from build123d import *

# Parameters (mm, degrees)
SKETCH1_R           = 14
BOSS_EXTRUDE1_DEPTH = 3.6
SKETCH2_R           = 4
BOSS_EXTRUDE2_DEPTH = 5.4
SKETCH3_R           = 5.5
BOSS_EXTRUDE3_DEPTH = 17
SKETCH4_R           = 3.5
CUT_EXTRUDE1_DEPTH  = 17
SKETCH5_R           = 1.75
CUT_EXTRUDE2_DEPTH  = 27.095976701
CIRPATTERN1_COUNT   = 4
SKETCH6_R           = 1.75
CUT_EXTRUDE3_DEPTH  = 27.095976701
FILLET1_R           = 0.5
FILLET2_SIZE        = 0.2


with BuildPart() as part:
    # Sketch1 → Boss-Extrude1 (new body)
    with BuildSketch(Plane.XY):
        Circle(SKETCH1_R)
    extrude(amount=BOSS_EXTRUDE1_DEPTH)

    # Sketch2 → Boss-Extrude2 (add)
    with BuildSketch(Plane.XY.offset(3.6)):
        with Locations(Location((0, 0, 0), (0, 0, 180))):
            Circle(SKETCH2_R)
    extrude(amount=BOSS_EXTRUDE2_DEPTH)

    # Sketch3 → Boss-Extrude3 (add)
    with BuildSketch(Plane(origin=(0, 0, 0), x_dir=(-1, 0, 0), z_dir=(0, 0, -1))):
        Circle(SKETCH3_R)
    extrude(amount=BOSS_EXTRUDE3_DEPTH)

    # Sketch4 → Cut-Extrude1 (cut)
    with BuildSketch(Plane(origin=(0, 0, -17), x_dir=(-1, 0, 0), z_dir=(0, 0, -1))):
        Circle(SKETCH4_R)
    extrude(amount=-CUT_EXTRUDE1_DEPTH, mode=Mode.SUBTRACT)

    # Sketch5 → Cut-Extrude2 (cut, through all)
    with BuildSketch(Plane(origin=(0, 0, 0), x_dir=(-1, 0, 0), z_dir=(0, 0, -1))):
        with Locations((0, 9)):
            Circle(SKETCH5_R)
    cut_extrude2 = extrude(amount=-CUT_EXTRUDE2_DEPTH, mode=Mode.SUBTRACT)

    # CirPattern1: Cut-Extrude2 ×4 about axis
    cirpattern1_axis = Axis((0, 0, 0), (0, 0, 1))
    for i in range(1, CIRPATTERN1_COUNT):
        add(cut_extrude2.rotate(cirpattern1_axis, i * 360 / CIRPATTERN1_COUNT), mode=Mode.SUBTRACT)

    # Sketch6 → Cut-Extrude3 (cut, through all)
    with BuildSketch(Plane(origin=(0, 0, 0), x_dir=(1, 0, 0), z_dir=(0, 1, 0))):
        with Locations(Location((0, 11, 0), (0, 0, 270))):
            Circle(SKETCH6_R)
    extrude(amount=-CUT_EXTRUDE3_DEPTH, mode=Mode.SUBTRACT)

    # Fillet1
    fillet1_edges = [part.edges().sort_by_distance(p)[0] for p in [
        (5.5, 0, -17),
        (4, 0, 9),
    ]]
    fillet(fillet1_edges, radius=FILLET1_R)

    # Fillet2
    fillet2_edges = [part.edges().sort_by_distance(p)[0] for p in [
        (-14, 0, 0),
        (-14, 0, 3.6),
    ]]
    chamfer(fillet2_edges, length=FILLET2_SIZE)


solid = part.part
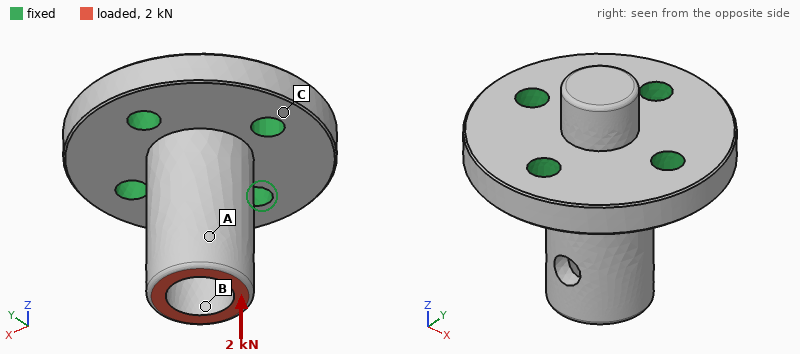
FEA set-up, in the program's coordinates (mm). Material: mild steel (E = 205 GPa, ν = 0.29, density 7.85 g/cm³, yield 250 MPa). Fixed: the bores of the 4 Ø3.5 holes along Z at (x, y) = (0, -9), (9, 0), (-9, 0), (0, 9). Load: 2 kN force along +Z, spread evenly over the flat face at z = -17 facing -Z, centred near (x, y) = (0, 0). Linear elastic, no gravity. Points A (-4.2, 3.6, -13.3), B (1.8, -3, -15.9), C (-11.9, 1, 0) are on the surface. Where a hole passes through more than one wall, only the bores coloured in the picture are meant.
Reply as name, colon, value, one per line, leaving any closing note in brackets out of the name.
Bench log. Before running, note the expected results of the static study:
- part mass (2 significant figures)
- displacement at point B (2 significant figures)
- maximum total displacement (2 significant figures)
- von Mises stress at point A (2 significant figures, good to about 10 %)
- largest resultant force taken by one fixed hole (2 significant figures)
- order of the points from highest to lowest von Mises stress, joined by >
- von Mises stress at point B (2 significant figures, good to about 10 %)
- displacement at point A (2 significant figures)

part mass: 26 g
displacement at point B: 4.8 µm
maximum total displacement: 5.2 µm
von Mises stress at point A: 30 MPa
largest resultant force taken by one fixed hole: 510 N
order of the points from highest to lowest von Mises stress, joined by >: B > A > C
von Mises stress at point B: 52 MPa
displacement at point A: 3.4 µm
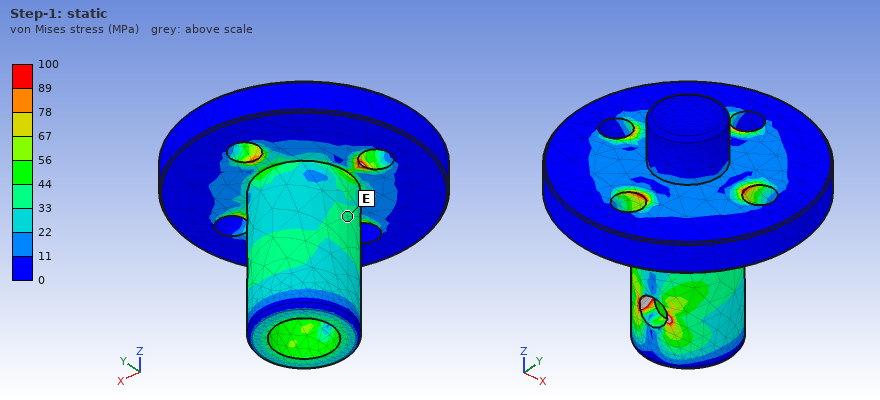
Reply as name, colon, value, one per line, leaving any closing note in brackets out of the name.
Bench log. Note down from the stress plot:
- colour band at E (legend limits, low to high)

colour band at E: 33 to 44 MPa
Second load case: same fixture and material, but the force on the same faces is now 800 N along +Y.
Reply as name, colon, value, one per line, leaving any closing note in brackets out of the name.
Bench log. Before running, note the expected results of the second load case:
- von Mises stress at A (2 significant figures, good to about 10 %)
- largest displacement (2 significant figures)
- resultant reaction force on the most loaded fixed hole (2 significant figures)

von Mises stress at A: 43 MPa
largest displacement: 26 µm
resultant reaction force on the most loaded fixed hole: 990 N
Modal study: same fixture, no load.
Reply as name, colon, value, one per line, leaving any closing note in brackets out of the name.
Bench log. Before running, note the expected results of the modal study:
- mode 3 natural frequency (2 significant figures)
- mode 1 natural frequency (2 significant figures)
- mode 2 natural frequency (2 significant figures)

mode 3 natural frequency: 43 kHz
mode 1 natural frequency: 19 kHz
mode 2 natural frequency: 19 kHz
